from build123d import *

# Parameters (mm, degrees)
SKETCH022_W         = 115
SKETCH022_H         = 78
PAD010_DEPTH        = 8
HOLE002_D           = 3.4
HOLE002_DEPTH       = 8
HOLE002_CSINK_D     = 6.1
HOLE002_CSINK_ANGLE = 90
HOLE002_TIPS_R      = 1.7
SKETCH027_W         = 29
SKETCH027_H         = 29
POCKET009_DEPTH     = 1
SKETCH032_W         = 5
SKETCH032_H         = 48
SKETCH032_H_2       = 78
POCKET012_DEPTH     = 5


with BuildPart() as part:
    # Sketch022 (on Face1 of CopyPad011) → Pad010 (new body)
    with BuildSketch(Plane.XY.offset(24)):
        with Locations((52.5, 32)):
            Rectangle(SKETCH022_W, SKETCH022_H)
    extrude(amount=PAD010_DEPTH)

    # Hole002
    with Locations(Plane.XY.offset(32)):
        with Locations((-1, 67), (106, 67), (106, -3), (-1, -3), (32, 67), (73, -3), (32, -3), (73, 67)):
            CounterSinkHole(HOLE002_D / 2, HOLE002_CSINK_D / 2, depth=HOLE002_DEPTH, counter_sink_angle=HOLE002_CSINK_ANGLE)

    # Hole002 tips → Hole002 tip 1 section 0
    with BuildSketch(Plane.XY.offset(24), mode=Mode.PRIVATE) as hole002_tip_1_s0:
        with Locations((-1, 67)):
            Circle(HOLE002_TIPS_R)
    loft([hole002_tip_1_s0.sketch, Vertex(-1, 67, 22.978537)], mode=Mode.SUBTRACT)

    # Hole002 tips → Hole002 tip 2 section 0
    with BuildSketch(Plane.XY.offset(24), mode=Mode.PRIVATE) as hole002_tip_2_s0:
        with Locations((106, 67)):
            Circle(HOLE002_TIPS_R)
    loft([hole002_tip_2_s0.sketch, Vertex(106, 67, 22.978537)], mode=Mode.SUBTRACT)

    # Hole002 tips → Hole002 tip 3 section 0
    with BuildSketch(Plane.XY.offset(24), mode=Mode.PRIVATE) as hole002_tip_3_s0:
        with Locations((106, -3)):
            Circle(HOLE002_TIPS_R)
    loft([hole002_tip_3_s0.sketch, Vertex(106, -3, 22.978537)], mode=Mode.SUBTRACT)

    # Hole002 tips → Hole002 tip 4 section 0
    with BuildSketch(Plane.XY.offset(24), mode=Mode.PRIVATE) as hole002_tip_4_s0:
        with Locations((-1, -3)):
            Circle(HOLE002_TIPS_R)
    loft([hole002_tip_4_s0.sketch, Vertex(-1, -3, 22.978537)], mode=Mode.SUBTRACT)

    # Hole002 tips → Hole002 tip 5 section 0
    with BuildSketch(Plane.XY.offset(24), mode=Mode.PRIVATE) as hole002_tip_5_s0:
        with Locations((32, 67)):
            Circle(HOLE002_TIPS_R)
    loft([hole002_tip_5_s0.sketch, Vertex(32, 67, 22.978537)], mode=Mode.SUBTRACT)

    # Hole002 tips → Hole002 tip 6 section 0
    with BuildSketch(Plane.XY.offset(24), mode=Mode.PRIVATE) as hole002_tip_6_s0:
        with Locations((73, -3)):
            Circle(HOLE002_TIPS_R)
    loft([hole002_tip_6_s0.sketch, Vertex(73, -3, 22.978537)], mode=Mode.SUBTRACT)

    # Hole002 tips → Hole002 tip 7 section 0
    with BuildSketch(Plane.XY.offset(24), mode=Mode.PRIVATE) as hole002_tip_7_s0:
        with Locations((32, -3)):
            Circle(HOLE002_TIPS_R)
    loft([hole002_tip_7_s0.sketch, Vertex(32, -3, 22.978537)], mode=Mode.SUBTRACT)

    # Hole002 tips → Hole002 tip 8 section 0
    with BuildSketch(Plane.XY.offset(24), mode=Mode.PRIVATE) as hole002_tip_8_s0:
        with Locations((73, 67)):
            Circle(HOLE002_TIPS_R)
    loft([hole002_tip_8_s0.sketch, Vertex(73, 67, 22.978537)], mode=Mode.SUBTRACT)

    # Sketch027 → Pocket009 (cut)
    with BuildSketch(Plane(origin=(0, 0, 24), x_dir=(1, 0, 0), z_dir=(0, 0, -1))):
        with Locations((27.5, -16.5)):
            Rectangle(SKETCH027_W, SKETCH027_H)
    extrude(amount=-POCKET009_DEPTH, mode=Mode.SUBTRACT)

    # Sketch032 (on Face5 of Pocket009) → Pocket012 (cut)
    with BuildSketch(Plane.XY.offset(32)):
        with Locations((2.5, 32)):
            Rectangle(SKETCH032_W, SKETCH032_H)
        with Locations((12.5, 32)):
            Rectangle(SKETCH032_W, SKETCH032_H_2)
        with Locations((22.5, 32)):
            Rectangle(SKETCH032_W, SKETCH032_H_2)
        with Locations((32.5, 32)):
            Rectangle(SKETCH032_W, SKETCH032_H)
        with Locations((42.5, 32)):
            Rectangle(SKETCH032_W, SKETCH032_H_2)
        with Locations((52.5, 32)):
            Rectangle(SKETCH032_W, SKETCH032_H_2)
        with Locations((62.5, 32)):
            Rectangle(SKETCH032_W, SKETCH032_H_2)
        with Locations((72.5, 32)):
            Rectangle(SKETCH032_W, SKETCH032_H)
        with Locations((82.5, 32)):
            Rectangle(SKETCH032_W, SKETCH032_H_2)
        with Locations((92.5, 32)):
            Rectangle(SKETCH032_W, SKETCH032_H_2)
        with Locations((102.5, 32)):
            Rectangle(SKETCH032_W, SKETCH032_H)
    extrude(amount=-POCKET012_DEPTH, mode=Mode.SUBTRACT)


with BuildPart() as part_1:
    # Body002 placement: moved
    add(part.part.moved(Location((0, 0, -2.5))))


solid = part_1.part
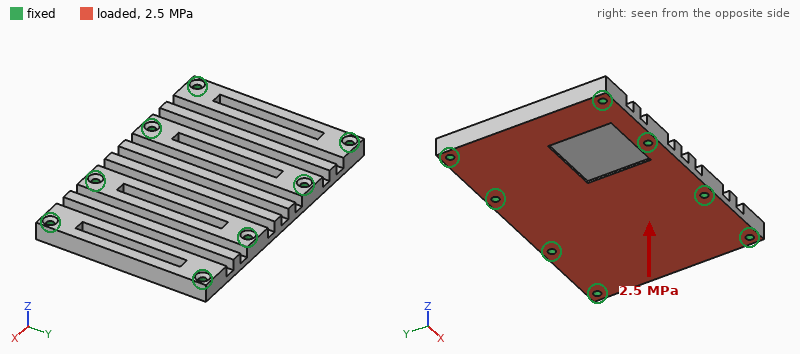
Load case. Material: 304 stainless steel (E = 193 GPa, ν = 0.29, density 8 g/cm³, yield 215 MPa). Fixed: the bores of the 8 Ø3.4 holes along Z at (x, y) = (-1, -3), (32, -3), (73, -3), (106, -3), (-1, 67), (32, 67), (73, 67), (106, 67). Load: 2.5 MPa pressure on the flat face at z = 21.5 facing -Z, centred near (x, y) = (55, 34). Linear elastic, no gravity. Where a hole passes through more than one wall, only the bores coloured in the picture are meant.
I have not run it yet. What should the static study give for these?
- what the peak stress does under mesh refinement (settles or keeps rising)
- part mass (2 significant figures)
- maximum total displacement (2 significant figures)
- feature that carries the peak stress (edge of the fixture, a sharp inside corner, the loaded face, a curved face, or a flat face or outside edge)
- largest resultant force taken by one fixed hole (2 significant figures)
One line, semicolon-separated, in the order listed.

keeps rising; 410 g; 58 µm; edge of the fixture; 3.6 kN
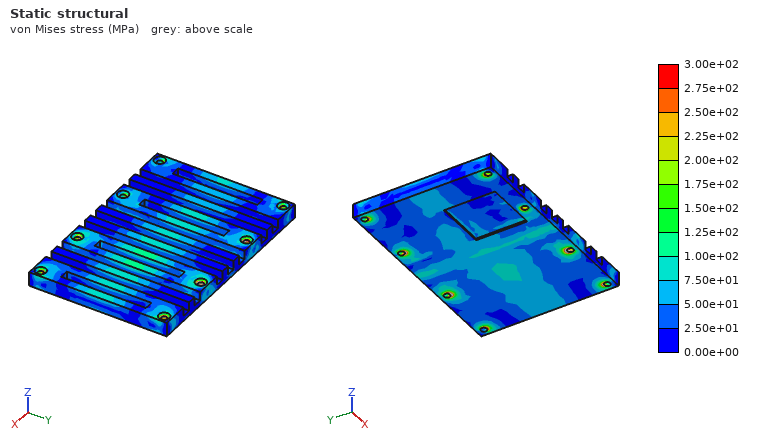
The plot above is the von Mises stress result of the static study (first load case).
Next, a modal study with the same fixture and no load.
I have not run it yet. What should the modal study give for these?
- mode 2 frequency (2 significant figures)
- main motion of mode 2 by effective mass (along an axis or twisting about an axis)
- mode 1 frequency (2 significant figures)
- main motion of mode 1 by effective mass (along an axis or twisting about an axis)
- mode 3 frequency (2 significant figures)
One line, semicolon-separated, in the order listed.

6500 Hz; twisting about Y; 5800 Hz; along Z; 6900 Hz
